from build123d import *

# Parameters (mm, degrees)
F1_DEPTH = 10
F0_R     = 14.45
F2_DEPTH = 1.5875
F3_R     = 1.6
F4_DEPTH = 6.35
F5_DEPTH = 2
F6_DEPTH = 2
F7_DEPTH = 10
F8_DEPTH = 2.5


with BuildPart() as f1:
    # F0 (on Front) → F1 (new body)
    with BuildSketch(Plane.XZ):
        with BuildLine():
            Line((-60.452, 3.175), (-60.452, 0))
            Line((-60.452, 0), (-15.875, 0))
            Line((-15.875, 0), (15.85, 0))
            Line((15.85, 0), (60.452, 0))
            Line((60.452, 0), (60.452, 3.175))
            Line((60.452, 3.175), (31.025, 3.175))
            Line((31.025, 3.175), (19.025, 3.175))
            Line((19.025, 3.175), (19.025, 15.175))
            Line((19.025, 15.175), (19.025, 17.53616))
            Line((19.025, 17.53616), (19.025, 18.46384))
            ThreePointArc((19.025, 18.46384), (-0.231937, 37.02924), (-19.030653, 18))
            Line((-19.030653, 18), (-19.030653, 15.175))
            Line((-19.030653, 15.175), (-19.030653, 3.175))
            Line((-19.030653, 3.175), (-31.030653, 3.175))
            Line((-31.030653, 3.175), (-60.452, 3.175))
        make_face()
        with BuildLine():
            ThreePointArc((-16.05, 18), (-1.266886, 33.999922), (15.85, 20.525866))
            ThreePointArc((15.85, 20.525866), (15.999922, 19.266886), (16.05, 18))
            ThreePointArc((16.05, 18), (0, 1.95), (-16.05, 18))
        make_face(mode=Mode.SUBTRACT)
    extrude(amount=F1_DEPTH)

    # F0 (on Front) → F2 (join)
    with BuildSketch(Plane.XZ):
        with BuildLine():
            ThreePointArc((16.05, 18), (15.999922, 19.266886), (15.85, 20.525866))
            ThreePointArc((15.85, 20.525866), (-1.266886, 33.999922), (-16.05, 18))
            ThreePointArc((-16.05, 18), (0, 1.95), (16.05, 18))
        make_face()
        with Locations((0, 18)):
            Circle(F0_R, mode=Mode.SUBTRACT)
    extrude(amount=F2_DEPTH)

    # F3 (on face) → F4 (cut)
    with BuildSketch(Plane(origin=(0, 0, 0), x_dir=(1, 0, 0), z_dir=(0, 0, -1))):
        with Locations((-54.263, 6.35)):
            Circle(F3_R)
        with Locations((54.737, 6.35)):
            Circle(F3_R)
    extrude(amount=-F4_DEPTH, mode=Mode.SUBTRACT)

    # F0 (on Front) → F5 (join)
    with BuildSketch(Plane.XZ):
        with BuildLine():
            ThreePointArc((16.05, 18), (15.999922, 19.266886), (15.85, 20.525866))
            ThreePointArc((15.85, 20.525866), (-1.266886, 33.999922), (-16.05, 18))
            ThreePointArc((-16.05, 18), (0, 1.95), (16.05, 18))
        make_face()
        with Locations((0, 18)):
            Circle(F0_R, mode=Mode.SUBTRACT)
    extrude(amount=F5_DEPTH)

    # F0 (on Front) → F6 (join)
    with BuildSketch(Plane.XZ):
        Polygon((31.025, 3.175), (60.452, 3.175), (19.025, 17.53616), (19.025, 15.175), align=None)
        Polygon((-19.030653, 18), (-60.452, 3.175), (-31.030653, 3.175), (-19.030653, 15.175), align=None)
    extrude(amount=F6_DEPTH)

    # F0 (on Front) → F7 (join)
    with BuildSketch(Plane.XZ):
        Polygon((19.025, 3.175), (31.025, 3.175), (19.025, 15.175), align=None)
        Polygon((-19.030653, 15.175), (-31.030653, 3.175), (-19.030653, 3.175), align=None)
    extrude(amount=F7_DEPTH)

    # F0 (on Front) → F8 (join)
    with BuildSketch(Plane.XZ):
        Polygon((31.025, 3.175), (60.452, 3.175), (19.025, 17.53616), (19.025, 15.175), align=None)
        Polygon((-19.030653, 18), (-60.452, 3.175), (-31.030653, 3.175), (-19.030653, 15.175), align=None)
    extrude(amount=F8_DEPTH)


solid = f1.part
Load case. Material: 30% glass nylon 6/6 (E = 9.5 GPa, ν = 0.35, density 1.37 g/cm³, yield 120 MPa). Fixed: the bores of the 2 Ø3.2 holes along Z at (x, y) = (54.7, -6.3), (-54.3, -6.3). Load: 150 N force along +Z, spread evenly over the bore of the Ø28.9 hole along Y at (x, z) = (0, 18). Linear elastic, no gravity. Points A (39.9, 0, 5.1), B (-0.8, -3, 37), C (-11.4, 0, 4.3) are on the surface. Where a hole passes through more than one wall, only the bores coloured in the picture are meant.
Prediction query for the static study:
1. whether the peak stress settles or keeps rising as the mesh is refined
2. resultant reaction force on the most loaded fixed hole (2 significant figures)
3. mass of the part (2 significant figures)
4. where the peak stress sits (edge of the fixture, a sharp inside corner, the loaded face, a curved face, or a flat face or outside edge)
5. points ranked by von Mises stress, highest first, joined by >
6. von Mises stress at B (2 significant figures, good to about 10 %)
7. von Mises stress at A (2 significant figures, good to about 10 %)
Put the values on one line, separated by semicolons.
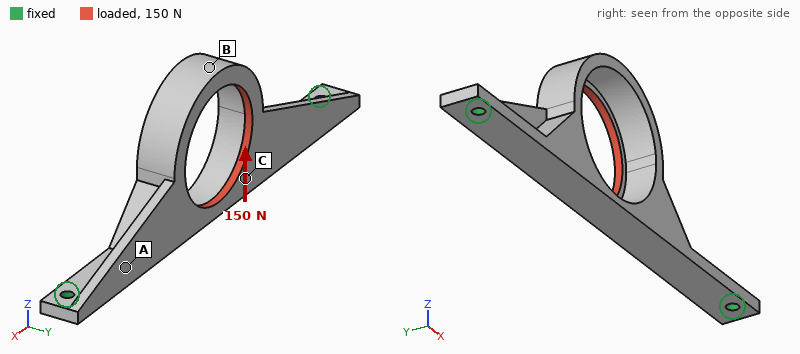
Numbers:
keeps rising; 90 N; 14 g; edge of the fixture; B > A > C; 13 MPa; 8.7 MPa
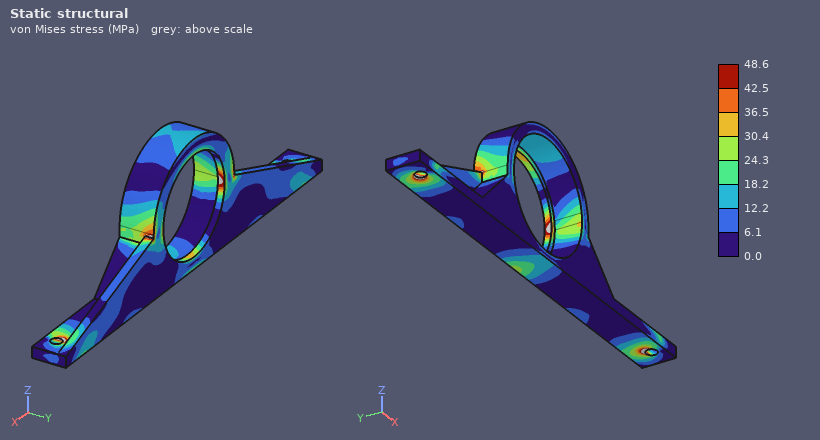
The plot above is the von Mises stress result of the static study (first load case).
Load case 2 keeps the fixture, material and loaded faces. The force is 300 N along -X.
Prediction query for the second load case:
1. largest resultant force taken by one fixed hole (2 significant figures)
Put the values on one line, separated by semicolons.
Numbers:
160 N
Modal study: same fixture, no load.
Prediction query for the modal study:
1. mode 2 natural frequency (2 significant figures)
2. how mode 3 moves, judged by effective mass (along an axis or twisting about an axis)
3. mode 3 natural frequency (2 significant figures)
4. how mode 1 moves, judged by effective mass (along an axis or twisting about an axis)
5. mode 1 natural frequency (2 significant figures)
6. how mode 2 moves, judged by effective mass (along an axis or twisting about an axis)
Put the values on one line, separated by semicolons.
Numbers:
990 Hz; along Y; 1700 Hz; along Y; 590 Hz; along Z
